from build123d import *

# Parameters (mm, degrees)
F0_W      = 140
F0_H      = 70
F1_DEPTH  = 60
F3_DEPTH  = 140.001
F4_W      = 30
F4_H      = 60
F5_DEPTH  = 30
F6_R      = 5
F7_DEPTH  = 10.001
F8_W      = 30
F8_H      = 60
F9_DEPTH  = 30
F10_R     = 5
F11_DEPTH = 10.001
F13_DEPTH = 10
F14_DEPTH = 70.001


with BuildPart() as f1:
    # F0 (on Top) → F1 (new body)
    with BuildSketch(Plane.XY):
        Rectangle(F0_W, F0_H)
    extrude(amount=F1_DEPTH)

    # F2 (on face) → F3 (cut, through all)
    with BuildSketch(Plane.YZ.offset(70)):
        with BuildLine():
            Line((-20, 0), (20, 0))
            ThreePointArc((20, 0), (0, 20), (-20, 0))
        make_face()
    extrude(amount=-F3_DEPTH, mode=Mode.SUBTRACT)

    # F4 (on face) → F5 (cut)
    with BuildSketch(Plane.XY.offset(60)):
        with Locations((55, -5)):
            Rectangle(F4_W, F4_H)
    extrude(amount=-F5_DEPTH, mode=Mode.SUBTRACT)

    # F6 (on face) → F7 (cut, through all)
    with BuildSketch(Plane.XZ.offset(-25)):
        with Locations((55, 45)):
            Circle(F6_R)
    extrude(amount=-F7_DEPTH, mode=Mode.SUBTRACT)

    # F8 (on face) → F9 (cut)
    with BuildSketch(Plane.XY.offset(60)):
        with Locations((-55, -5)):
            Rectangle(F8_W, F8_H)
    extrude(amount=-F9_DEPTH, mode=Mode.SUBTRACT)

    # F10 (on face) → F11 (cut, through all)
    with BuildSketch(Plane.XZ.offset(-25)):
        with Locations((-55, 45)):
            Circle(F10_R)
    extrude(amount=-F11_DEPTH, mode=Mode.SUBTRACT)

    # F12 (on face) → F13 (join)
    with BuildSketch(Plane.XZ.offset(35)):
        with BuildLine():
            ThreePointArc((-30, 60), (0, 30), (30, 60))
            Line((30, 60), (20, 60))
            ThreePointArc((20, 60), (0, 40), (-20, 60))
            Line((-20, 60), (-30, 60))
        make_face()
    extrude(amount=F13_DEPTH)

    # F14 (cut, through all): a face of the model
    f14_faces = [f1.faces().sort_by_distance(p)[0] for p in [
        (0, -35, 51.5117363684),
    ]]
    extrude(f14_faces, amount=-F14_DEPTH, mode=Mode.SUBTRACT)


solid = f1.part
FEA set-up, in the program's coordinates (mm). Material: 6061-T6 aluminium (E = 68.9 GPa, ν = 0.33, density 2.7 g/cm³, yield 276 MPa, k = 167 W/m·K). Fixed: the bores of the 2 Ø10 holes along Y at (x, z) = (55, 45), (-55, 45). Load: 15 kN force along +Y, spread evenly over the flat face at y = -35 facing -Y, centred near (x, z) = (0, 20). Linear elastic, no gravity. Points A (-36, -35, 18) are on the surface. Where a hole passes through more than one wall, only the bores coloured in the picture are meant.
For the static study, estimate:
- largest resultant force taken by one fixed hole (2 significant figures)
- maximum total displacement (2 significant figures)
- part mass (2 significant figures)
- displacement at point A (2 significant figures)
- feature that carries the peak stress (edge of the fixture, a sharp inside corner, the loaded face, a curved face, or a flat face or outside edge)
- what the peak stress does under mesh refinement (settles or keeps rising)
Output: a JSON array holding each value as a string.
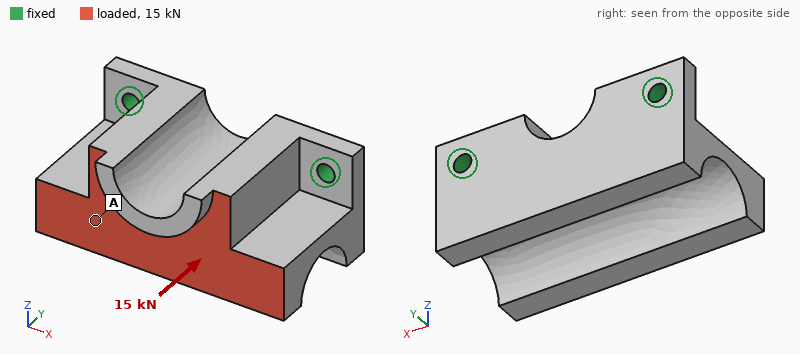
["7.6 kN", "0.43 mm", "960 g", "0.37 mm", "edge of the fixture", "keeps rising"]
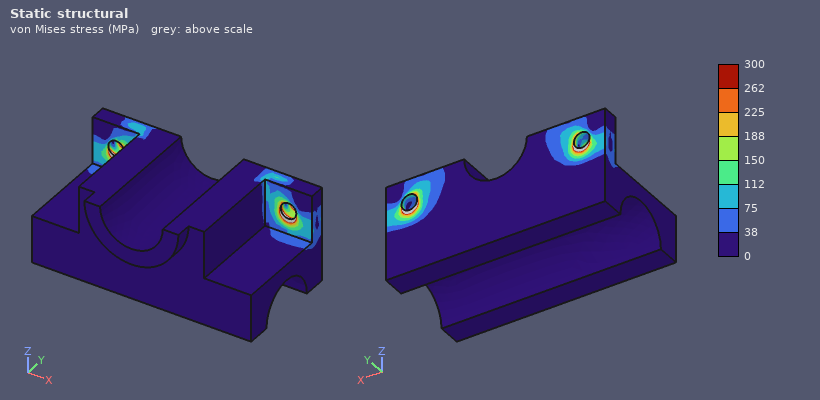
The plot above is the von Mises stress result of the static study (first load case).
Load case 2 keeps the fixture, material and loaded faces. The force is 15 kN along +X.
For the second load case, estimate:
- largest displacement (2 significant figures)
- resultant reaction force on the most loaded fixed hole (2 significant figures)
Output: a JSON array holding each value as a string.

["80 µm", "12 kN"]
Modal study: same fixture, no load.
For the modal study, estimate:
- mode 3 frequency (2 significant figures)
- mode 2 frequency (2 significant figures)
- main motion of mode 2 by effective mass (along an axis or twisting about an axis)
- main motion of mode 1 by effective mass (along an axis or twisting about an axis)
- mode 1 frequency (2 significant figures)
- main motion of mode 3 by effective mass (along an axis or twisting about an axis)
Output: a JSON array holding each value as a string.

["3900 Hz", "3400 Hz", "along X", "along Z", "920 Hz", "along X"]
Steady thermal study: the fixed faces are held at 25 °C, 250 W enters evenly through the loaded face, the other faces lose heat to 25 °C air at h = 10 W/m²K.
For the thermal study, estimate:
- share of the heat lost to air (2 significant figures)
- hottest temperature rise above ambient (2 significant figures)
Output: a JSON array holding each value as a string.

["6.3 %", "57 K"]
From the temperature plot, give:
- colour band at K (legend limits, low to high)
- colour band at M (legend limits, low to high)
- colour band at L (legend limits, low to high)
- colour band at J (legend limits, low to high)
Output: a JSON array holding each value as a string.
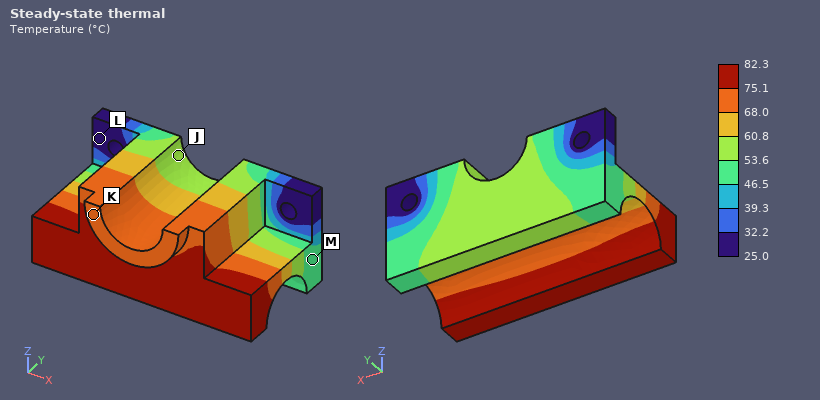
["68.0 to 75.1 °C", "46.5 to 53.6 °C", "25.0 to 32.2 °C", "53.6 to 60.8 °C"]
